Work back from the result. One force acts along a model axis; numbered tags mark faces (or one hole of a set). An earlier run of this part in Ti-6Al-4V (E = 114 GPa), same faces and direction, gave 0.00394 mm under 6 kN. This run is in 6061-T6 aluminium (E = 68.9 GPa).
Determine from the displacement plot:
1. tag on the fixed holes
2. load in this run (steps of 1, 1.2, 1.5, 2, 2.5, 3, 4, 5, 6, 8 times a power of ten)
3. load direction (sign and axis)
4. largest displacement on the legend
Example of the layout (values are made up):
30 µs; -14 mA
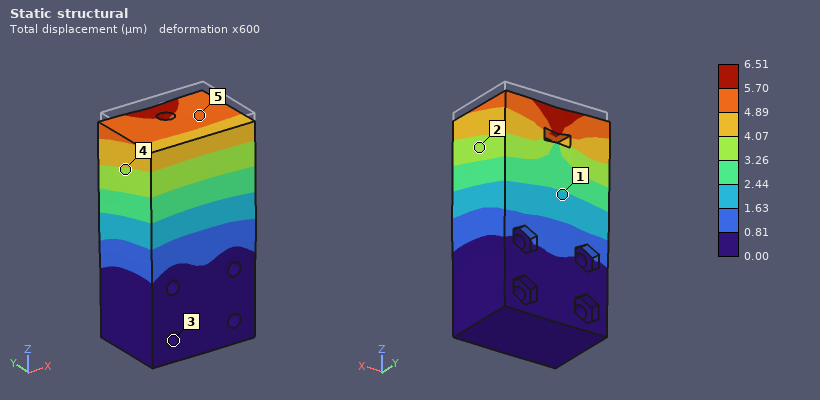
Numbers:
3; 6 kN; -Z; 6.51 µm
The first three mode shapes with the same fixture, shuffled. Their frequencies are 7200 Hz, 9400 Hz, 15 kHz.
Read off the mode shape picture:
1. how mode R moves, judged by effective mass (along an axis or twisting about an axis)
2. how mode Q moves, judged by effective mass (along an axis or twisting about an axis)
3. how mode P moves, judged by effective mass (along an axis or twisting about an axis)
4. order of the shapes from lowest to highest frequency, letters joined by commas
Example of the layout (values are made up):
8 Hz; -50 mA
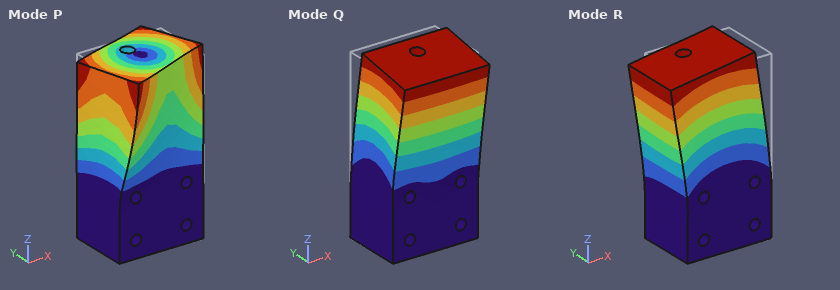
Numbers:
along X; along Y; twisting about Z; Q, R, P
